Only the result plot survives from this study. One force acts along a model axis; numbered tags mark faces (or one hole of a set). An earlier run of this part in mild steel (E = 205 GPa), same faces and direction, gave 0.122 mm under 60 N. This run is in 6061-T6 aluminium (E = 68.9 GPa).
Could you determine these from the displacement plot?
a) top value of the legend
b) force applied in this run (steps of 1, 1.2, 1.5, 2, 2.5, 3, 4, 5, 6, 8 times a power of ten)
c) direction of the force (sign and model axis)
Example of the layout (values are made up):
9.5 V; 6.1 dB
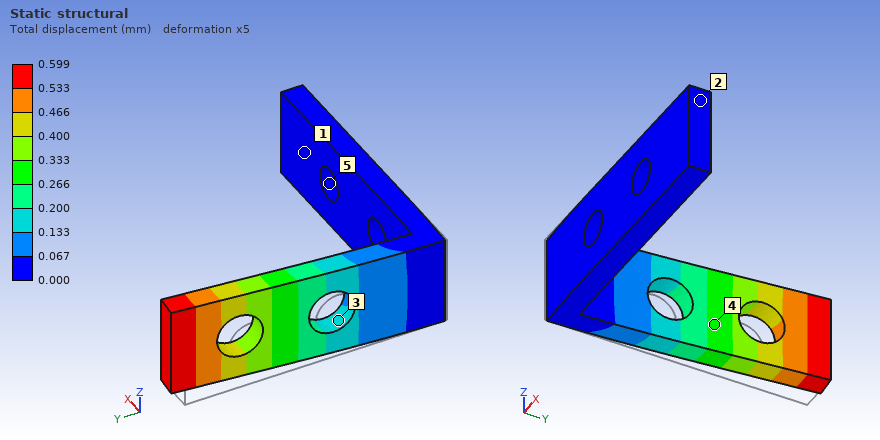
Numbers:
0.599 mm; 100 N; +X
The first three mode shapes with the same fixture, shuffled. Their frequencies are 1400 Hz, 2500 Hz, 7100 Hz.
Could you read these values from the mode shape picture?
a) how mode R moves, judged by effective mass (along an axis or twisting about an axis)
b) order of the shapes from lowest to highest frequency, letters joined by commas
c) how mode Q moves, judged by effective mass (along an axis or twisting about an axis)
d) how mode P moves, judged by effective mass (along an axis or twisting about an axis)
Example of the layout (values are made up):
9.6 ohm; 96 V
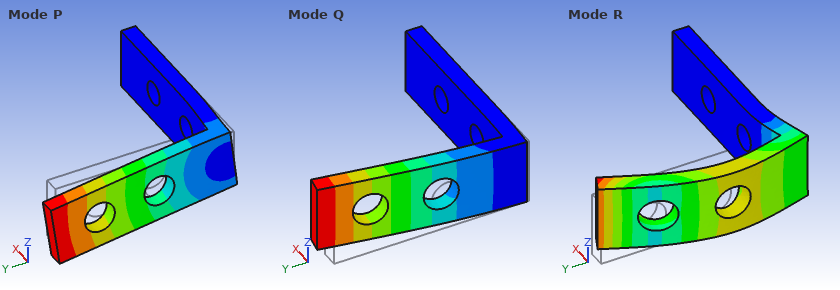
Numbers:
along Y; Q, P, R; along X; along Z
